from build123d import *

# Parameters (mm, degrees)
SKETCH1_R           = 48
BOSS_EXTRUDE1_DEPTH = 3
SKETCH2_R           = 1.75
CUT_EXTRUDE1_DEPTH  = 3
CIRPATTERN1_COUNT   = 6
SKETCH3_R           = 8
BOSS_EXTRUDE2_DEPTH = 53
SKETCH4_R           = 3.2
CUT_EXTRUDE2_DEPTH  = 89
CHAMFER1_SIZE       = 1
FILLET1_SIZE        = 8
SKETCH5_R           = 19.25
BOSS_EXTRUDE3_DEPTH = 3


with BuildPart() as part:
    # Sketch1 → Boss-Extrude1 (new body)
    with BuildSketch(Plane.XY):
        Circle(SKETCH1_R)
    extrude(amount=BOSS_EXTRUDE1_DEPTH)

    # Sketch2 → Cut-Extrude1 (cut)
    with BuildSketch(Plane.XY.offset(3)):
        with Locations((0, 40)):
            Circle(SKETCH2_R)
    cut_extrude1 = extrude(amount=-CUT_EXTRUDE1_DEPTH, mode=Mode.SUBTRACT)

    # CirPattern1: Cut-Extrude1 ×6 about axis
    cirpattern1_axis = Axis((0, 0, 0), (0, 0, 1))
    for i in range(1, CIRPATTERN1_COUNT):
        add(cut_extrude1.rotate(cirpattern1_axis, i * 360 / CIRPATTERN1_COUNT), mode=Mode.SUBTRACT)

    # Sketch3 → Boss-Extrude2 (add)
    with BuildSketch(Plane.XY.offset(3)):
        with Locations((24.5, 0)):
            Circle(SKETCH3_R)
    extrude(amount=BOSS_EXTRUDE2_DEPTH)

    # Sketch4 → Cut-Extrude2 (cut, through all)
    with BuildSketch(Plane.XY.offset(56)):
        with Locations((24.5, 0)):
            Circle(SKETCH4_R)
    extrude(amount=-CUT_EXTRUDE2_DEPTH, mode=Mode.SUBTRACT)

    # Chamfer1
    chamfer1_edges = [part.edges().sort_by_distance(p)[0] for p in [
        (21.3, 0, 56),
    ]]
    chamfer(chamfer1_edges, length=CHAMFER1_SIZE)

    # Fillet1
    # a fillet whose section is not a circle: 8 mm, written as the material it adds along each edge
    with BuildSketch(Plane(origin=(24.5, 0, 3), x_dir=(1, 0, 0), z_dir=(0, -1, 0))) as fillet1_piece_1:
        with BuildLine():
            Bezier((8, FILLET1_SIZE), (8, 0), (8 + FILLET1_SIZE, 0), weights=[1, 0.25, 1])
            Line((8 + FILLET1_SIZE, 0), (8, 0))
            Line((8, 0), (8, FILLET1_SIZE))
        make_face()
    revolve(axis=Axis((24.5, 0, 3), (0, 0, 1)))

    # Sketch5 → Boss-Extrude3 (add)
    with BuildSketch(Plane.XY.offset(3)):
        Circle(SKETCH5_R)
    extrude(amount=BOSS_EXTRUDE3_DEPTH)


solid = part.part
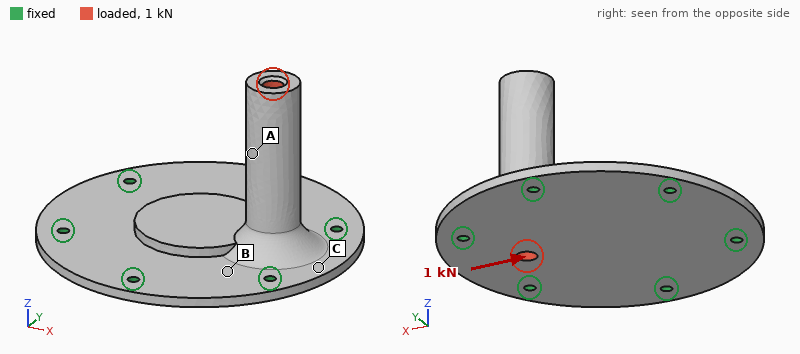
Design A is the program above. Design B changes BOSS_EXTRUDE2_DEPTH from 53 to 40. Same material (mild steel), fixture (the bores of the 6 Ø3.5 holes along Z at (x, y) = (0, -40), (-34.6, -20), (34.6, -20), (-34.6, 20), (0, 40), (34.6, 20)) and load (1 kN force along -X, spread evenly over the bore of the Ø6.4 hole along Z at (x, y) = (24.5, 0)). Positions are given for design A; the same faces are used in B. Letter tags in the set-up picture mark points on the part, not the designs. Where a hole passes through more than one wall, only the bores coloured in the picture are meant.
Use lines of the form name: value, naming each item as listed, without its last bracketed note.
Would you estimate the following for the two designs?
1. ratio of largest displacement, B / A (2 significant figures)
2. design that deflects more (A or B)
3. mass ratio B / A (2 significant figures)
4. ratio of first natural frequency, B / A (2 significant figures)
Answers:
ratio of largest displacement, B / A: 0.53
design that deflects more: A
mass ratio B / A: 0.94
ratio of first natural frequency, B / A: 1.4
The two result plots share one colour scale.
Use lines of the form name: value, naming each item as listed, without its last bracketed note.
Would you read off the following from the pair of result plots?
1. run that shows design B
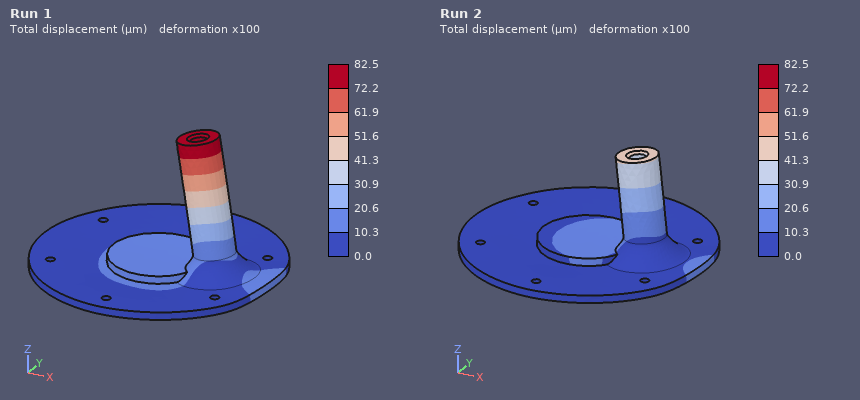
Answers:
run that shows design B: Run 2
